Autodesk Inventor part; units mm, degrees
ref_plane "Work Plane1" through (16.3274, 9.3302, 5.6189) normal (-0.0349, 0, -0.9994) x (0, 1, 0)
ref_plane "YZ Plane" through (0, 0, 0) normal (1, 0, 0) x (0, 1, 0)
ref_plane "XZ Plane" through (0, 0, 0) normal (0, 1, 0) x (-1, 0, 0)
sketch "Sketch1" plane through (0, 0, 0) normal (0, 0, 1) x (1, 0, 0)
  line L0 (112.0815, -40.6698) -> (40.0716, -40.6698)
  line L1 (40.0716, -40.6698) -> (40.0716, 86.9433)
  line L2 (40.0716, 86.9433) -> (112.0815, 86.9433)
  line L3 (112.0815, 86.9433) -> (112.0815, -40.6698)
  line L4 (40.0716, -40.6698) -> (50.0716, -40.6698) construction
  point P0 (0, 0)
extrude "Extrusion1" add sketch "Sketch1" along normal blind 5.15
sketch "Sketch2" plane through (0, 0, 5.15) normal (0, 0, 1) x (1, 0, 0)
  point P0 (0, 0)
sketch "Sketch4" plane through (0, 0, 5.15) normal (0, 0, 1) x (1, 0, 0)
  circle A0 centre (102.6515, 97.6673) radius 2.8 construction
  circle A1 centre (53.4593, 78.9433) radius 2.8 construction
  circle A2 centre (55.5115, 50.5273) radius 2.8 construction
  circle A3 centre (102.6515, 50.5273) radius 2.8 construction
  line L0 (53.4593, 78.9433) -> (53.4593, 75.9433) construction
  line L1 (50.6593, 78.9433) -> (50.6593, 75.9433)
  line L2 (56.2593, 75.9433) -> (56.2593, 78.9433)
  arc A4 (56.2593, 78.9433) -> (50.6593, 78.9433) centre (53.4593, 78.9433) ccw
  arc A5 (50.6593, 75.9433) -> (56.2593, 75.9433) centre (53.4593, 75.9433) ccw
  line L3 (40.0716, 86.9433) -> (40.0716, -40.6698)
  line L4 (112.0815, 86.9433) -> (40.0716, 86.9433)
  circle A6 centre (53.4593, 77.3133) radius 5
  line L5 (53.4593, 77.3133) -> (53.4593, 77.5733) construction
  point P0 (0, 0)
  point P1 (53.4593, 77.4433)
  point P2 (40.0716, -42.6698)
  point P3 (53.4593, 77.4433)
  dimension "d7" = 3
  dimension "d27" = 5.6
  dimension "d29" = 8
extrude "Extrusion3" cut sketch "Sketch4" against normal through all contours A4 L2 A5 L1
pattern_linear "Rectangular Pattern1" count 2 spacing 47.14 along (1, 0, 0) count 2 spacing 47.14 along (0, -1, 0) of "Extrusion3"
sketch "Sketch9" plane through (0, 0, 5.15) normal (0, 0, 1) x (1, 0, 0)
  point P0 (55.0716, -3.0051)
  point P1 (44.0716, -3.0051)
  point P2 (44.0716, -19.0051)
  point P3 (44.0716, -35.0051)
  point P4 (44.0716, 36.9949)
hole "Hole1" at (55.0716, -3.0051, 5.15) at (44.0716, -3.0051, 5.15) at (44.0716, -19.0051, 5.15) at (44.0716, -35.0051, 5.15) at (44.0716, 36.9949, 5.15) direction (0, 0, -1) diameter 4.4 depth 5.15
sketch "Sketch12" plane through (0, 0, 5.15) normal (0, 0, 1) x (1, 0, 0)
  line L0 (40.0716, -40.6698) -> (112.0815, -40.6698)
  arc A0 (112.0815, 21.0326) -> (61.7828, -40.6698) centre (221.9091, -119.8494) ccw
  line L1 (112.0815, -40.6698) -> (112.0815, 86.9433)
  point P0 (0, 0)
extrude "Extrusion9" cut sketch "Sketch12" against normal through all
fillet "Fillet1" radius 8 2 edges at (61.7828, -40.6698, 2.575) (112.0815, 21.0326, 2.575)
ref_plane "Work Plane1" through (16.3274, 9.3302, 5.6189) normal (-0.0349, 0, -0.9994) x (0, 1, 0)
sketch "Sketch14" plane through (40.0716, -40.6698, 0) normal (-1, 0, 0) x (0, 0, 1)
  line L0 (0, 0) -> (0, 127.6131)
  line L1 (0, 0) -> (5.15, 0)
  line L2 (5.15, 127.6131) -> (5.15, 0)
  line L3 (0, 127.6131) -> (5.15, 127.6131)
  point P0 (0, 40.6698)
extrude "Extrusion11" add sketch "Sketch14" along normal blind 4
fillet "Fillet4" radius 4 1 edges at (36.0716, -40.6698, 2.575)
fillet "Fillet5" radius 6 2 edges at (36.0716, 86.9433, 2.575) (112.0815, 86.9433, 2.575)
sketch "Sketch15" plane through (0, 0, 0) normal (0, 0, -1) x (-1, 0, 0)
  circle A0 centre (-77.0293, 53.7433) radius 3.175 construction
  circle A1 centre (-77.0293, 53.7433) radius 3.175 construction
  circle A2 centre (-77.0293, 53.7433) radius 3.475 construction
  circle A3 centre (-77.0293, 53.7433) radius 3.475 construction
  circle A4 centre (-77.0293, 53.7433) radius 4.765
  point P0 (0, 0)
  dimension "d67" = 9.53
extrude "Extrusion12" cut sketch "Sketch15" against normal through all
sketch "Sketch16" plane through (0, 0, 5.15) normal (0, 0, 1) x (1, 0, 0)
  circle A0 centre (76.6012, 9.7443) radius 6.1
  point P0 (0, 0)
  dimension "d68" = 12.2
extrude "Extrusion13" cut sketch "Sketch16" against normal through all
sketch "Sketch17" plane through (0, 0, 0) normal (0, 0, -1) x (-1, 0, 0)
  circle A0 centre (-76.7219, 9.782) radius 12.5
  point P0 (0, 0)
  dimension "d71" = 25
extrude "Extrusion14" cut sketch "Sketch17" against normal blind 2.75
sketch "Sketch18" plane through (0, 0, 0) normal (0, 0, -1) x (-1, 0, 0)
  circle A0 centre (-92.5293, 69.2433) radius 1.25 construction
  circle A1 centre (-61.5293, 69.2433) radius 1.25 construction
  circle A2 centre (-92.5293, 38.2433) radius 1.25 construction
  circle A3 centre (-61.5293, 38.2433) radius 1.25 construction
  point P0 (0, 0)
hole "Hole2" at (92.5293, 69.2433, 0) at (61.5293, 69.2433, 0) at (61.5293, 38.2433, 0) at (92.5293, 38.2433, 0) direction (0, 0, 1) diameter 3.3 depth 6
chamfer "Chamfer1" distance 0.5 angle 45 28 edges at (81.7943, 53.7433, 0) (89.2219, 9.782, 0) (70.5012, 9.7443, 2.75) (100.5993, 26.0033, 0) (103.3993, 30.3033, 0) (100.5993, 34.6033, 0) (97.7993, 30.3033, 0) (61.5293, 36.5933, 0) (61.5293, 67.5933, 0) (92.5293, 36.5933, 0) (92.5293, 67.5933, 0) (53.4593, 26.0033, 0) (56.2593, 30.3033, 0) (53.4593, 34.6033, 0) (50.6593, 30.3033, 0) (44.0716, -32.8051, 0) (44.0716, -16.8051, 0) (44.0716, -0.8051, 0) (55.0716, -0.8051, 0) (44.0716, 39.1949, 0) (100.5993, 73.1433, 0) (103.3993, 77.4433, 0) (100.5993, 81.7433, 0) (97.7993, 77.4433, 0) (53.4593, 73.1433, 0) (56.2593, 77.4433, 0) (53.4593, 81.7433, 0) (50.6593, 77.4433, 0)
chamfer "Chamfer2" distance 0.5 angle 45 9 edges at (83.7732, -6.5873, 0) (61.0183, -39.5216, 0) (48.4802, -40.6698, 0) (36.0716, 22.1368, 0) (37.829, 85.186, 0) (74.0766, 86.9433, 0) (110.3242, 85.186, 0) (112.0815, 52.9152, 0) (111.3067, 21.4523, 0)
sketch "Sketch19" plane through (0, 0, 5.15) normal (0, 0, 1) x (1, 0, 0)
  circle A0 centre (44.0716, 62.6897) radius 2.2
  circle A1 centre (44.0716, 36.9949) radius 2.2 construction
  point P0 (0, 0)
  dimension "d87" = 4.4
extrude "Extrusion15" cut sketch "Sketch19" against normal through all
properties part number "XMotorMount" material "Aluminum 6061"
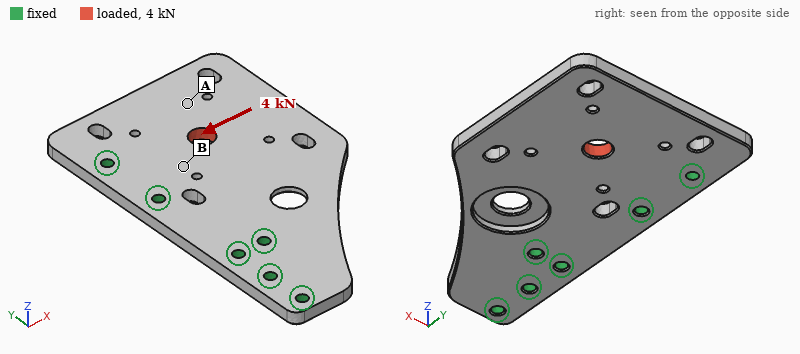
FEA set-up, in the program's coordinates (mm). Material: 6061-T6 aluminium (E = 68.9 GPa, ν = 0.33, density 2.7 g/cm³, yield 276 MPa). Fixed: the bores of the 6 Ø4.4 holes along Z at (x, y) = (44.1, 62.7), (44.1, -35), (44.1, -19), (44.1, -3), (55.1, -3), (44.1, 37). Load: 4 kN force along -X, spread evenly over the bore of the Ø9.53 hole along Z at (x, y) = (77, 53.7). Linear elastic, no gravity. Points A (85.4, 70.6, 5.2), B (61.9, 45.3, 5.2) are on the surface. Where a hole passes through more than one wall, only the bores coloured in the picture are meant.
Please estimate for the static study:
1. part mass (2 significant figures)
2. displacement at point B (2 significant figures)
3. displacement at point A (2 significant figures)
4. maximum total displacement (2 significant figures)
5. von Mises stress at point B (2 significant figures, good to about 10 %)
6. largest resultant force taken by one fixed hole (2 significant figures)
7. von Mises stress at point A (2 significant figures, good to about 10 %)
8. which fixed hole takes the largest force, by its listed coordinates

100 g
7.0 µm
20 µm
34 µm
21 MPa
2.6 kN
6.3 MPa
(44.1, 62.7)
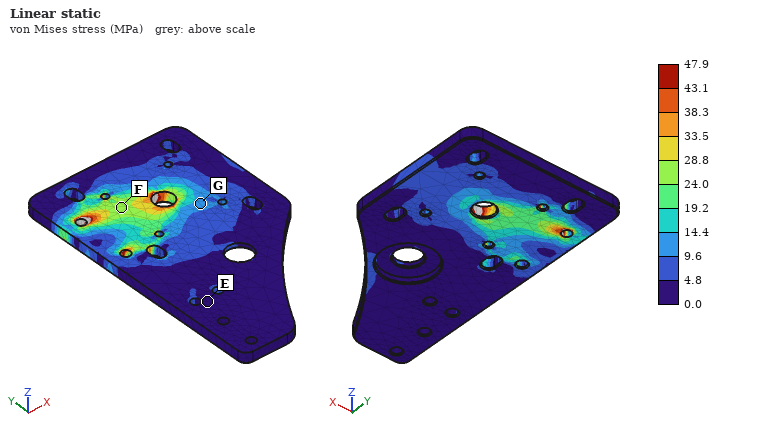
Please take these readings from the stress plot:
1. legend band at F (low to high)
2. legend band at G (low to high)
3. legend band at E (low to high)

24.0 to 28.8 MPa
9.6 to 14.4 MPa
0.0 to 4.8 MPa
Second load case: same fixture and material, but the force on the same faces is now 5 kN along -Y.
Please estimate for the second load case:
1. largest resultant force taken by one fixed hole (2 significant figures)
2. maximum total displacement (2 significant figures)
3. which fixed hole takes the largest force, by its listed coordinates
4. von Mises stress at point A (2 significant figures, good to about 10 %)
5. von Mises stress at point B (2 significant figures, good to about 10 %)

2.6 kN
34 µm
(44.1, 62.7)
9.0 MPa
30 MPa
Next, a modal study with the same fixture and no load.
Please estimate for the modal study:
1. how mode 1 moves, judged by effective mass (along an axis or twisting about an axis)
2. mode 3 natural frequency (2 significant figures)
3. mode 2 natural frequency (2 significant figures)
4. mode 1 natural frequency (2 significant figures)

along Z
4800 Hz
2300 Hz
960 Hz
